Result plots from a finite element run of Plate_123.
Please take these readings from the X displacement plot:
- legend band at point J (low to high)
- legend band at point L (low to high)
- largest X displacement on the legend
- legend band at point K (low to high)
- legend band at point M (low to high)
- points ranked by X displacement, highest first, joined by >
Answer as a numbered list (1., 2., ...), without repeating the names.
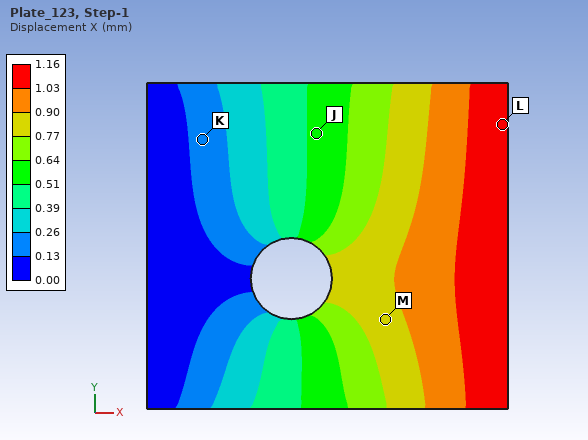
1. 0.51 to 0.64 mm
2. 1.03 to 1.16 mm
3. 1.16 mm
4. 0.13 to 0.26 mm
5. 0.77 to 0.90 mm
6. L > M > J > K
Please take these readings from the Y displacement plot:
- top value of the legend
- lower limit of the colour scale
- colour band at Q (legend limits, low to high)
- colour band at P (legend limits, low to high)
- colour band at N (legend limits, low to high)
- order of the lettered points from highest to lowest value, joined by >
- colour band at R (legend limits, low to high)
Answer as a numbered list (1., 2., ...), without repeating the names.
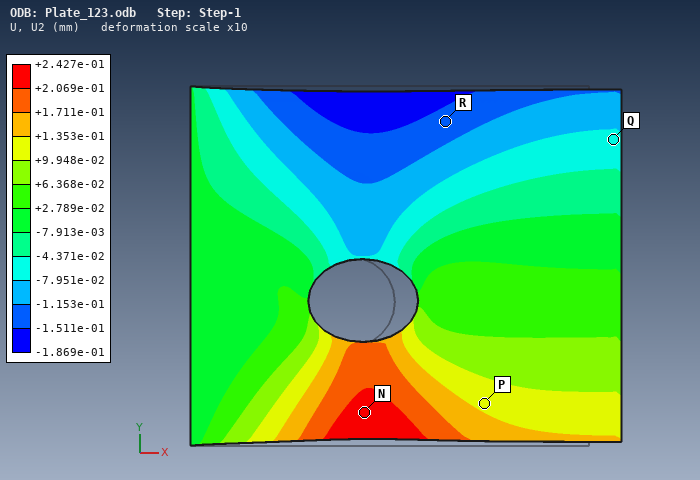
1. +2.427e-01 mm
2. -1.869e-01 mm
3. -7.951e-02 to -4.371e-02 mm
4. +9.948e-02 to +1.353e-01 mm
5. +2.069e-01 to +2.427e-01 mm
6. N > P > Q > R
7. -1.511e-01 to -1.153e-01 mm
